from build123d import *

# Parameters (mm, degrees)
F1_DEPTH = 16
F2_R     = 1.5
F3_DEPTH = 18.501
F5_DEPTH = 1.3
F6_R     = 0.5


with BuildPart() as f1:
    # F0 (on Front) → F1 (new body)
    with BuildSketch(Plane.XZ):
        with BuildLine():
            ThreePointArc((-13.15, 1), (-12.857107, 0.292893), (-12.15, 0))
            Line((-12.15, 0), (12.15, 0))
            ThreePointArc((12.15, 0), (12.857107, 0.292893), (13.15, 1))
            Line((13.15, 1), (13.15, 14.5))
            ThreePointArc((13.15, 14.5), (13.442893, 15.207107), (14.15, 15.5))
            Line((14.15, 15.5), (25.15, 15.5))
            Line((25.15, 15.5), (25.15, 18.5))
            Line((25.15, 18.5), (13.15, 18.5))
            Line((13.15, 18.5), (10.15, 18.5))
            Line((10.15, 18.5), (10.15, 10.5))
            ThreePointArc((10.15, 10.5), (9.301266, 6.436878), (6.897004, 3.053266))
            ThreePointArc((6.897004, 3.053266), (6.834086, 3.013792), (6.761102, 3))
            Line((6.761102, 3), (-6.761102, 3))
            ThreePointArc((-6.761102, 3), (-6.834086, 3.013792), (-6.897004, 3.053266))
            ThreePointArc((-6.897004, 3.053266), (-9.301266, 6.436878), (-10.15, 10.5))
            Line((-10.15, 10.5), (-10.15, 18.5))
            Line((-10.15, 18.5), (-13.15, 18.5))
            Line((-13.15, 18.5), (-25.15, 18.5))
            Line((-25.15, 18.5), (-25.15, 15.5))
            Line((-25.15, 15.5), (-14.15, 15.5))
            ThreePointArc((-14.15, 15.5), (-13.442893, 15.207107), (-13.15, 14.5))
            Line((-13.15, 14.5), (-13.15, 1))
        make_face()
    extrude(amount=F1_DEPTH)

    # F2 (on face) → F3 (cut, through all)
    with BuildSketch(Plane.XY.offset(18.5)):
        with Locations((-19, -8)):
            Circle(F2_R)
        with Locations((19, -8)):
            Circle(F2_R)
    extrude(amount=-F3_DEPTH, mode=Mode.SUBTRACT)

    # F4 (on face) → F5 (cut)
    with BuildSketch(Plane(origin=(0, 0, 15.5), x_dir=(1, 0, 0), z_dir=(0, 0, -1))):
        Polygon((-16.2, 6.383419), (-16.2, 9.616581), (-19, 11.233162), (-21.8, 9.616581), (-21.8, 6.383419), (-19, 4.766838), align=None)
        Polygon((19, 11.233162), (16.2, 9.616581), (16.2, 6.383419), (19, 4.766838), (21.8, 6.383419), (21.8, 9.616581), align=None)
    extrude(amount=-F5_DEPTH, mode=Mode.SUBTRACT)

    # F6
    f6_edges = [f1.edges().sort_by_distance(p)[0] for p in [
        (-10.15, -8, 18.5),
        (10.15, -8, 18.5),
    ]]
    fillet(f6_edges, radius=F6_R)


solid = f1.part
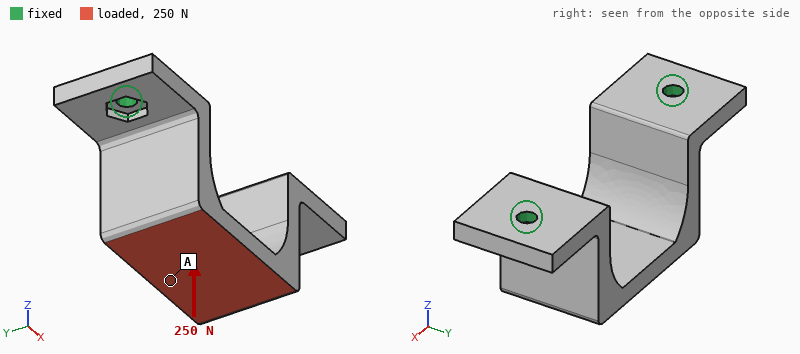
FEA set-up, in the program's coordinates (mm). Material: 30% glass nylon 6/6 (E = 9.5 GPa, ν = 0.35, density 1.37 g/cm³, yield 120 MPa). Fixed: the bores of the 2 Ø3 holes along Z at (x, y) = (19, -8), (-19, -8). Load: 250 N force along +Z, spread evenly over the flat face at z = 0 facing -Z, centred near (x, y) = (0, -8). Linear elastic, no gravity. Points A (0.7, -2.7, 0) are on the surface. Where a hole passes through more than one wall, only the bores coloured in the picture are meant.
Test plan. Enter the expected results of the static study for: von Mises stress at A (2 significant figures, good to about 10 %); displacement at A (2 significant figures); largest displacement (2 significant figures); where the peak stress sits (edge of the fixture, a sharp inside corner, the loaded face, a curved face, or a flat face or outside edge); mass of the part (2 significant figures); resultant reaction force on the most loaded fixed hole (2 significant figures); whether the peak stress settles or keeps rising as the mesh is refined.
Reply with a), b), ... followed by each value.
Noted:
a) 6.0 MPa
b) 48 µm
c) 49 µm
d) edge of the fixture
e) 5.5 g
f) 140 N
g) keeps rising
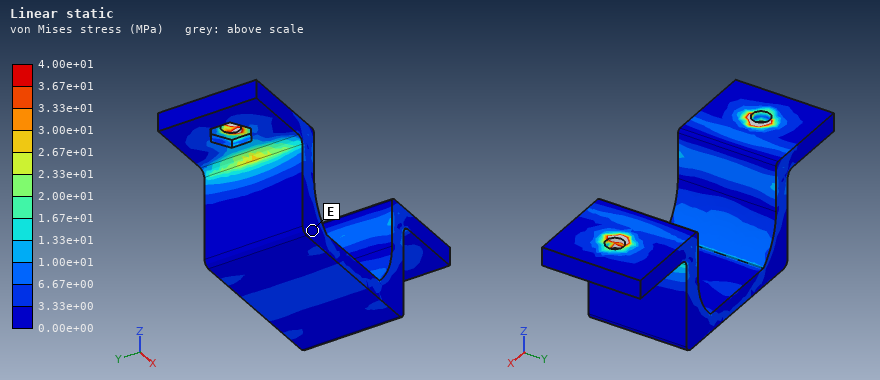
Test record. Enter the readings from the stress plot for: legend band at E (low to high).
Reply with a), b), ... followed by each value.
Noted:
a) 0.00e+00 to 3.33e+00 MPa
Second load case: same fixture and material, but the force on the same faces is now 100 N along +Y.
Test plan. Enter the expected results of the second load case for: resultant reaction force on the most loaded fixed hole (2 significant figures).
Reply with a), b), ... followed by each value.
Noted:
a) 50 N
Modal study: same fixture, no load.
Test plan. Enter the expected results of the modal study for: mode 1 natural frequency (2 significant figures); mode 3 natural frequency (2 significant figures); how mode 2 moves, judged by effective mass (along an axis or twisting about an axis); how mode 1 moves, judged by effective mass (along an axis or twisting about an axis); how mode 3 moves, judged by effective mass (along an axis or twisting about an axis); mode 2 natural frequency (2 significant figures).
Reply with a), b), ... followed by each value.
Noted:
a) 1700 Hz
b) 4700 Hz
c) along X
d) along Y
e) twisting about Z
f) 4200 Hz
